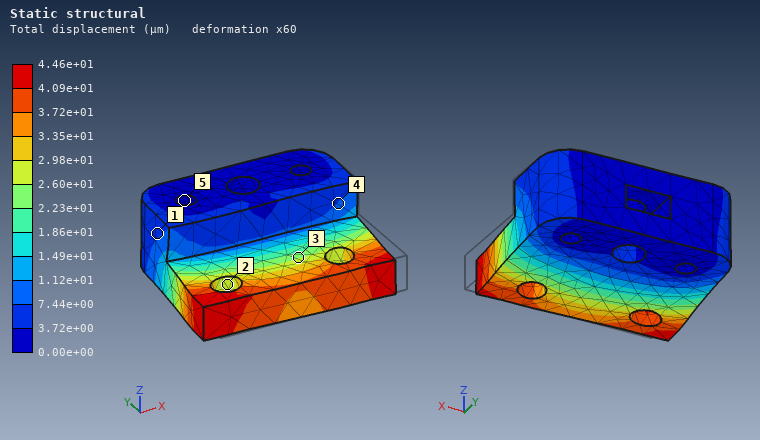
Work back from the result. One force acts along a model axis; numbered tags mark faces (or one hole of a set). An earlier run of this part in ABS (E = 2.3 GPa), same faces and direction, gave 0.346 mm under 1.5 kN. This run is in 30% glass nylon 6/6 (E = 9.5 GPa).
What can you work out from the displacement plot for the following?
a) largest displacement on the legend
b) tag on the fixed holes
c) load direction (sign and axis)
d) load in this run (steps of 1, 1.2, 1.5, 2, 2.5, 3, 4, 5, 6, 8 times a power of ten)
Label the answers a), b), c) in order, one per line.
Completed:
a) 4.46e+01 µm
b) 5
c) -X
d) 800 N
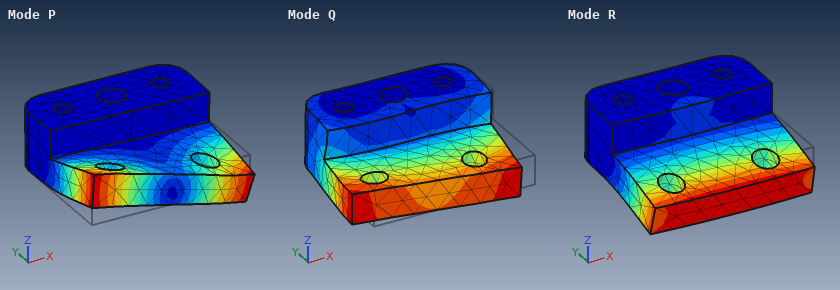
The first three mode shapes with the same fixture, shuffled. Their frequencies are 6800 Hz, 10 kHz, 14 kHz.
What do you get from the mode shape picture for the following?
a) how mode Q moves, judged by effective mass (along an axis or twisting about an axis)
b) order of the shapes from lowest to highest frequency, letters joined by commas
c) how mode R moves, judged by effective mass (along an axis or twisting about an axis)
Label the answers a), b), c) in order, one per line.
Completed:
a) along X
b) R, P, Q
c) along Z
